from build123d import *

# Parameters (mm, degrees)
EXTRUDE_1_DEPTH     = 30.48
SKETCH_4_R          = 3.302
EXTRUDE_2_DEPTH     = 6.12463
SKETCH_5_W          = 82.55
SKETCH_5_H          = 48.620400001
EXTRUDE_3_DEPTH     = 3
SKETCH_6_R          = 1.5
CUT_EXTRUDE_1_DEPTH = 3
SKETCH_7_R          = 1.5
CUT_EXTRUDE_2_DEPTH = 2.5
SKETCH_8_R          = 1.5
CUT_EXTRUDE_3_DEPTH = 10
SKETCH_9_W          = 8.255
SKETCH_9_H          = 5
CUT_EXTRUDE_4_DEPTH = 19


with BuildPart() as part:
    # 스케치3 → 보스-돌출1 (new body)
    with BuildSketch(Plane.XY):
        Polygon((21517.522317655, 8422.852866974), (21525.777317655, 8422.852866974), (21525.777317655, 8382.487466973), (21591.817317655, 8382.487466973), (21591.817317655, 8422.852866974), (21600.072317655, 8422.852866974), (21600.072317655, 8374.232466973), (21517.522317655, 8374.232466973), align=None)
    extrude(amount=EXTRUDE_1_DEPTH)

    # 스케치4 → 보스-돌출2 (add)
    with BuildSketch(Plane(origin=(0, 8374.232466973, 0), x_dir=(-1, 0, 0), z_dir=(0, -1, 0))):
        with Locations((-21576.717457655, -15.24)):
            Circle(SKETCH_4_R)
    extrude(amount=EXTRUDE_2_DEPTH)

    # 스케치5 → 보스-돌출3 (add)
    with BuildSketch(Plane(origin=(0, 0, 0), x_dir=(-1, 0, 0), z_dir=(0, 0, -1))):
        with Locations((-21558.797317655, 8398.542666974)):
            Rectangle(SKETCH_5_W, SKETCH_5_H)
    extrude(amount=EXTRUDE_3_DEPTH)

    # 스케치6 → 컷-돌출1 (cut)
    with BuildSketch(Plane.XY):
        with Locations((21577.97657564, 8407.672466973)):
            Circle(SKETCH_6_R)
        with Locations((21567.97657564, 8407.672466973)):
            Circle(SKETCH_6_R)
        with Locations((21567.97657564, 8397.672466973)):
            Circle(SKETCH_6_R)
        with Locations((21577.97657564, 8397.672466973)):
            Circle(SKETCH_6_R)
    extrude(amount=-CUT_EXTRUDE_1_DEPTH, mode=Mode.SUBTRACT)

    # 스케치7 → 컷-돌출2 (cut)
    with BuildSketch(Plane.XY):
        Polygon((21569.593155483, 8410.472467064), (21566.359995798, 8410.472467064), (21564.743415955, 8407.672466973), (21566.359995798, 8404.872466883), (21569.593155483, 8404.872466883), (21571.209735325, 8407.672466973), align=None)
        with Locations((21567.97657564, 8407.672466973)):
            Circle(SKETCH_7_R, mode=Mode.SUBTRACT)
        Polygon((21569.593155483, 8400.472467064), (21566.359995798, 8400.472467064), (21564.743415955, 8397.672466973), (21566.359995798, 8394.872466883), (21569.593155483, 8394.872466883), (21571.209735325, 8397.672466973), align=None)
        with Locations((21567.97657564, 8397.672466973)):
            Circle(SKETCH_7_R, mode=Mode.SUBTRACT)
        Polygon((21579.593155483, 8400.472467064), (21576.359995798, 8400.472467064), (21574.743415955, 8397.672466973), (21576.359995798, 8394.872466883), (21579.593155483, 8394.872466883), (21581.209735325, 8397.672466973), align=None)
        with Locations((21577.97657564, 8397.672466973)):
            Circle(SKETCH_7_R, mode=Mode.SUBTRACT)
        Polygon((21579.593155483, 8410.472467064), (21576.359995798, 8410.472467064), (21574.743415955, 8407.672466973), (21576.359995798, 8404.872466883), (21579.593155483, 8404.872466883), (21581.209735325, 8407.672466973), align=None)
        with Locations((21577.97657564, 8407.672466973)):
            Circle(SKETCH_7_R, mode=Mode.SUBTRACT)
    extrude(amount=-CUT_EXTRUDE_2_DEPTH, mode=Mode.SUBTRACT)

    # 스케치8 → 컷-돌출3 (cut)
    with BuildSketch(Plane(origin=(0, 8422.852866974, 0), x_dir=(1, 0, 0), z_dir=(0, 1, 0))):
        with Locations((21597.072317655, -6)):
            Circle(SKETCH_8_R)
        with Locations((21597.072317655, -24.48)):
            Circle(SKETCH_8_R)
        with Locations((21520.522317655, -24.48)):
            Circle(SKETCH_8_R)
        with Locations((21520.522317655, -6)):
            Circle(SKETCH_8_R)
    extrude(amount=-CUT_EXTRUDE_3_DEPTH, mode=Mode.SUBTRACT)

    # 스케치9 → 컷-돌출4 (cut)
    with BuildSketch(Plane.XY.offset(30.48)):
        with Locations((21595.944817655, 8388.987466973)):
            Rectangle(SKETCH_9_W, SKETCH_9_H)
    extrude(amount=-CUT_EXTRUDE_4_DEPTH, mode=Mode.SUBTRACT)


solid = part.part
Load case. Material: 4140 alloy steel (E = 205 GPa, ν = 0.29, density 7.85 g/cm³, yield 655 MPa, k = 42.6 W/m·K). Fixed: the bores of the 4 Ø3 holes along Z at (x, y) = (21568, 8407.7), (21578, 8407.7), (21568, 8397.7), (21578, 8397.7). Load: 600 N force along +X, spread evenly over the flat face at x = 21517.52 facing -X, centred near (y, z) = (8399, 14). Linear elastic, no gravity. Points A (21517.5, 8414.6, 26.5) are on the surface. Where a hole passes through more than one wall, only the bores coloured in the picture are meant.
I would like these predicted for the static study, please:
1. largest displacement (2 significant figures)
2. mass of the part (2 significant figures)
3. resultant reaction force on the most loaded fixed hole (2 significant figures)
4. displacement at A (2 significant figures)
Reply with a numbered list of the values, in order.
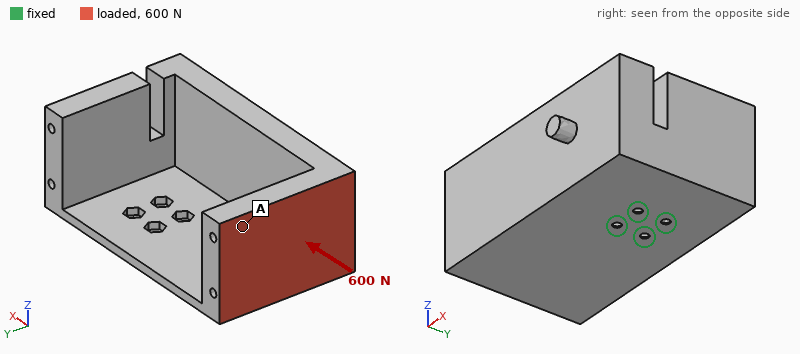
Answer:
1. 0.18 mm
2. 410 g
3. 600 N
4. 0.18 mm
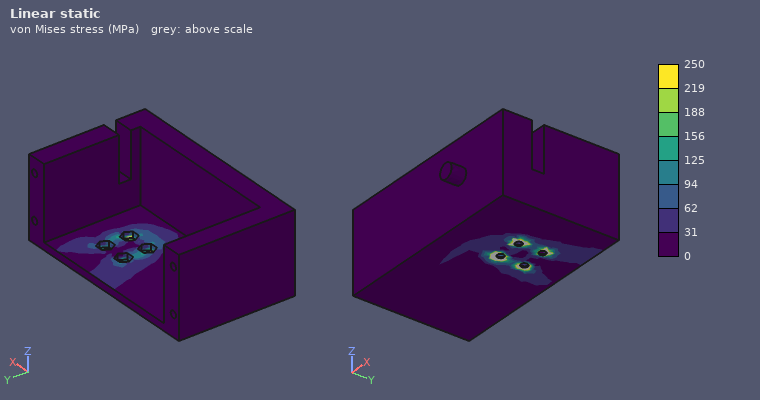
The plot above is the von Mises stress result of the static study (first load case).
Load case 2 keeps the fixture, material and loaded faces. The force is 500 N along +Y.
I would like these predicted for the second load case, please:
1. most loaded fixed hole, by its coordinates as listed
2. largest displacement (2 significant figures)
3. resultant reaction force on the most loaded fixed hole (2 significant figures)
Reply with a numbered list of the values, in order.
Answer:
1. (21568, 8407.7)
2. 0.15 mm
3. 1.2 kN
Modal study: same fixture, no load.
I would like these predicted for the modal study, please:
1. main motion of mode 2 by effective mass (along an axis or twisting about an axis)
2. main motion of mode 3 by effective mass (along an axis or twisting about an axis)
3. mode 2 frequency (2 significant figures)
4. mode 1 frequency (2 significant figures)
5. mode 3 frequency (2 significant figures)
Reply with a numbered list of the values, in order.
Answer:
1. along Y
2. along Z
3. 610 Hz
4. 400 Hz
5. 1600 Hz
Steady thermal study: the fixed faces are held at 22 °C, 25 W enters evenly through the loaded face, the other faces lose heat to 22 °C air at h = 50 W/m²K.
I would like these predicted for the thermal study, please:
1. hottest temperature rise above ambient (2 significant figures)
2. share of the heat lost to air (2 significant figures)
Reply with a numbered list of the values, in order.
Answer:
1. 61 K
2. 83 %
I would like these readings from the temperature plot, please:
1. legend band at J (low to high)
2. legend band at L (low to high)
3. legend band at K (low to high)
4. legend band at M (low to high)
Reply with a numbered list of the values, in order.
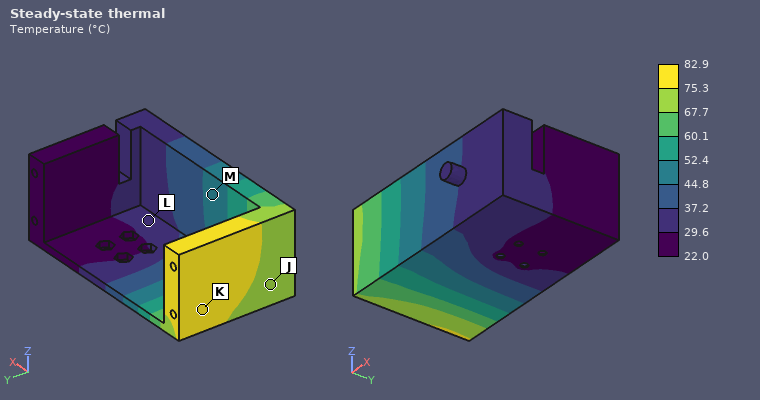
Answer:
1. 67.7 to 75.3 °C
2. 29.6 to 37.2 °C
3. 75.3 to 82.9 °C
4. 44.8 to 52.4 °C
